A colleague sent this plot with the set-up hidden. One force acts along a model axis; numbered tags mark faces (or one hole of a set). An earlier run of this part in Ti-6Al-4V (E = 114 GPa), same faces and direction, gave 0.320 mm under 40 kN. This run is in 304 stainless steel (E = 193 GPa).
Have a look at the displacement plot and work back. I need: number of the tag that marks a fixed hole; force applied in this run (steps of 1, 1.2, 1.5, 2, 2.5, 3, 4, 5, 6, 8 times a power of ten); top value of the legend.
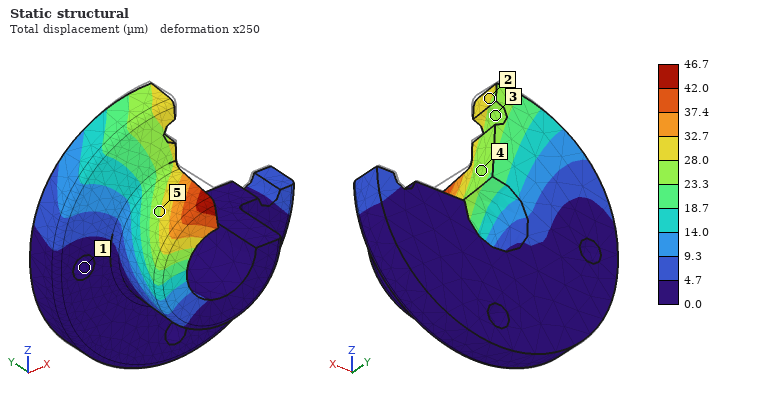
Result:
1
10 kN
46.7 µm
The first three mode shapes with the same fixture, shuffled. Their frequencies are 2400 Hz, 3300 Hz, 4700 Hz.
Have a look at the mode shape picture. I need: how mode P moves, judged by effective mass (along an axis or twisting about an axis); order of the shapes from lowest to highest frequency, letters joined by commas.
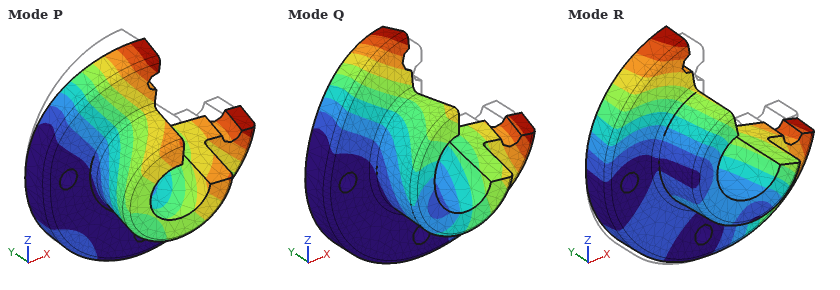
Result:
along Y
P, Q, R
